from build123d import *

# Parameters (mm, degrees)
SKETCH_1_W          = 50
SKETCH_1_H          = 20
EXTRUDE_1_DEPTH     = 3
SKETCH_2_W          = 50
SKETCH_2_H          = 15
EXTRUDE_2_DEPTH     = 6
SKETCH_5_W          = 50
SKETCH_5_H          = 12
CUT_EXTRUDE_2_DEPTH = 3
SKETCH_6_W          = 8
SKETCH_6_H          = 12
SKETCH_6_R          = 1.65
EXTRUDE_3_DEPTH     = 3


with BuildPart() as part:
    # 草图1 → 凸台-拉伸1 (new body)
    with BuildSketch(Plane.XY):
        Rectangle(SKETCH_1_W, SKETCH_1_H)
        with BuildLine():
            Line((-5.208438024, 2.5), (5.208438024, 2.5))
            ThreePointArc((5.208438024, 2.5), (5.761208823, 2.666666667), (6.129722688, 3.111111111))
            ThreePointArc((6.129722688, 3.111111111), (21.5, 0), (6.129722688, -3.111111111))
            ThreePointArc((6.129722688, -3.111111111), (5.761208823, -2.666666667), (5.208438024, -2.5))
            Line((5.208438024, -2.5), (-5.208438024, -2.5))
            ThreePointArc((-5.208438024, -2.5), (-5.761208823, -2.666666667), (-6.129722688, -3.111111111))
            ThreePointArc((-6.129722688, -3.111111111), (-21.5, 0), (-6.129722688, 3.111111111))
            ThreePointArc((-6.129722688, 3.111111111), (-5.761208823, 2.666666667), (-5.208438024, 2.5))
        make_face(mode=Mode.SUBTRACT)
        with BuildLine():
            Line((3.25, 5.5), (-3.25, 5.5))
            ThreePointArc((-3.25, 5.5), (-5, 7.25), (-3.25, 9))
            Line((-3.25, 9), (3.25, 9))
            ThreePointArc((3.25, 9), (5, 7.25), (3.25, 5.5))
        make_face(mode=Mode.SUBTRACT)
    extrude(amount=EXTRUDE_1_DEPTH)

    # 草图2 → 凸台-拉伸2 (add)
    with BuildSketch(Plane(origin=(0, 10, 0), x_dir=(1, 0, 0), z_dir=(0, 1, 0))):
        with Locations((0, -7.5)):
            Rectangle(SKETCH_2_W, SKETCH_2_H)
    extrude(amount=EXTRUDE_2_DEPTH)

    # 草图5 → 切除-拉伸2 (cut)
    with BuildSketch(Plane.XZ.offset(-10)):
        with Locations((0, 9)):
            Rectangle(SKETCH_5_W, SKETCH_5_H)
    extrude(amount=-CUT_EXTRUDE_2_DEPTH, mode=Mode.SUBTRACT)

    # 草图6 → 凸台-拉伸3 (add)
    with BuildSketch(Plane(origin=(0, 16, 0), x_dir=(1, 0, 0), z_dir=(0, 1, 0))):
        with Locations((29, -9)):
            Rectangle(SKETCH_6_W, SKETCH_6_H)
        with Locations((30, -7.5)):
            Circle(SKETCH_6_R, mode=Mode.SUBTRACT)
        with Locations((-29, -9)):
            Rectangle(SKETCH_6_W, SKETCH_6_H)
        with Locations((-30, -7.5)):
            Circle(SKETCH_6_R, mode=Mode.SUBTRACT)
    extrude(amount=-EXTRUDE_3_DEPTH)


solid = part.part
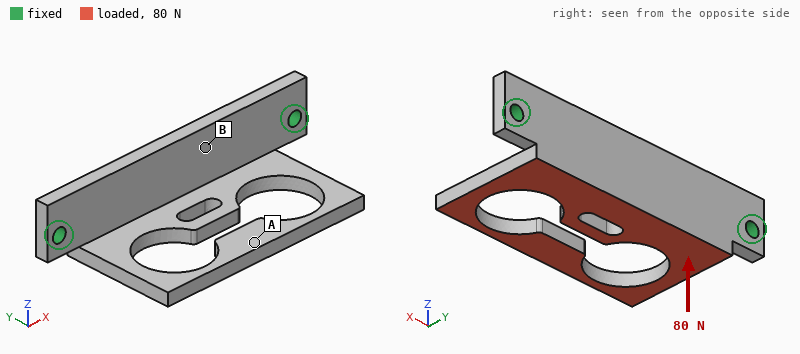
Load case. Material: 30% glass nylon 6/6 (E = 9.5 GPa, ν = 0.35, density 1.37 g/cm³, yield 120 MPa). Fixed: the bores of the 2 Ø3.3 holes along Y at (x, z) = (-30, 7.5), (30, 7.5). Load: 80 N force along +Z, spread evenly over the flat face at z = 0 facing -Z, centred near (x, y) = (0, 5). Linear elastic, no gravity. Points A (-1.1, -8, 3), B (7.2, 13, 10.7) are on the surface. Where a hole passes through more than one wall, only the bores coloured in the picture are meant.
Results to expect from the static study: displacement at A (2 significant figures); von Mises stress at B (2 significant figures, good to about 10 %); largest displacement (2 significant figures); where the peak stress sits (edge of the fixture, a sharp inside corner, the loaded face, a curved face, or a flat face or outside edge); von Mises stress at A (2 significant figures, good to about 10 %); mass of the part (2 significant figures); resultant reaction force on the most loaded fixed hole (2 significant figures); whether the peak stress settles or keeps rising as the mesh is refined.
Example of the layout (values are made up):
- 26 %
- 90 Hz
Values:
- 0.80 mm
- 3.4 MPa
- 0.86 mm
- edge of the fixture
- 8.2 MPa
- 6.5 g
- 40 N
- keeps rising
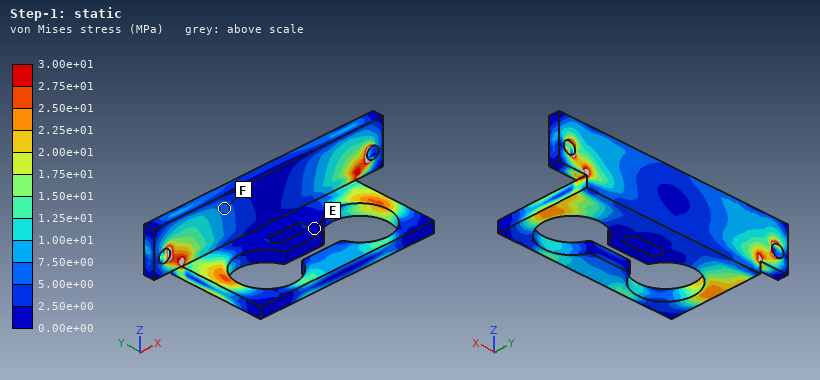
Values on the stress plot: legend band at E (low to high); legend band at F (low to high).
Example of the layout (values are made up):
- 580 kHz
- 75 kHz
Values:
- 0.00e+00 to 2.50e+00 MPa
- 5.00e+00 to 7.50e+00 MPa
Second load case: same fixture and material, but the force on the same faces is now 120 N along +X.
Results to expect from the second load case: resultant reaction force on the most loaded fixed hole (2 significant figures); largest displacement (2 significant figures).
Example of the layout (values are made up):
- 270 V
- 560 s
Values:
- 66 N
- 0.19 mm
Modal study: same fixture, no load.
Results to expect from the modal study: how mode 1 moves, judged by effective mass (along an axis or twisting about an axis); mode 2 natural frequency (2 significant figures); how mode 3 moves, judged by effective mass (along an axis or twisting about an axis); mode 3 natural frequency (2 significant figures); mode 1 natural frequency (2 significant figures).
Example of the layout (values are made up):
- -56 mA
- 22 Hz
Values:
- along Z
- 2100 Hz
- along X
- 2500 Hz
- 990 Hz
